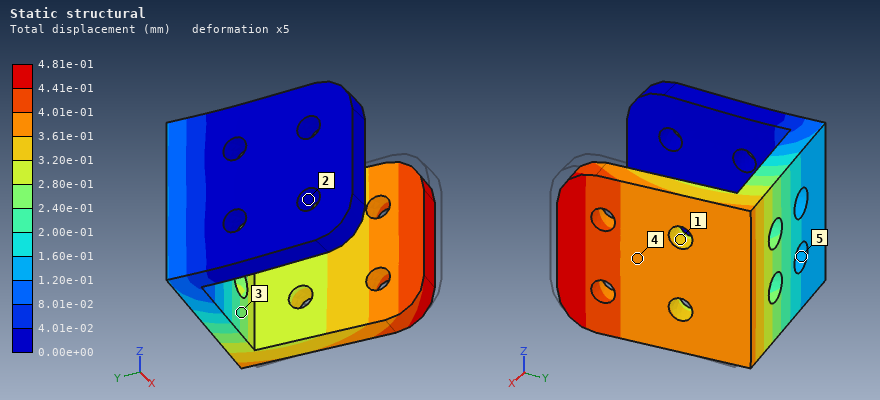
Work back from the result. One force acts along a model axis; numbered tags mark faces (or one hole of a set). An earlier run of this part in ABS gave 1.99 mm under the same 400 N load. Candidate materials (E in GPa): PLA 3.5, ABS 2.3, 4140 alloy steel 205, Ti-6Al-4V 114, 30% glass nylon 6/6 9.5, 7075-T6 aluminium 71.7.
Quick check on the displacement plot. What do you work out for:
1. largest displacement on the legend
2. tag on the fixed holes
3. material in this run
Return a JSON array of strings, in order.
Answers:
["4.81e-01 mm", "2", "30% glass nylon 6/6"]
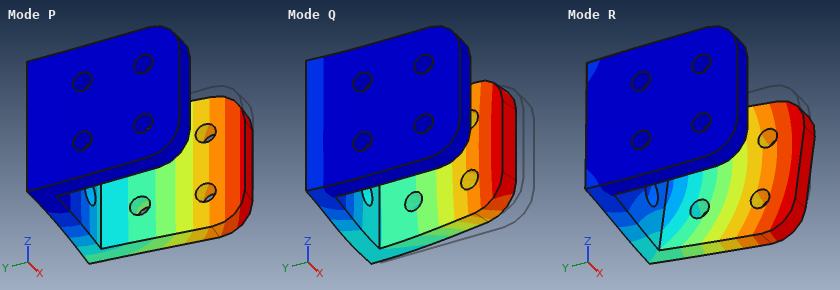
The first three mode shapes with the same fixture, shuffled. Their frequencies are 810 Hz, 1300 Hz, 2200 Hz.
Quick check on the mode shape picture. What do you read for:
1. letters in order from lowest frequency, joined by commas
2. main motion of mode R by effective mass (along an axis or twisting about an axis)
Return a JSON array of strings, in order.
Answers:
["P, R, Q", "along Z"]
